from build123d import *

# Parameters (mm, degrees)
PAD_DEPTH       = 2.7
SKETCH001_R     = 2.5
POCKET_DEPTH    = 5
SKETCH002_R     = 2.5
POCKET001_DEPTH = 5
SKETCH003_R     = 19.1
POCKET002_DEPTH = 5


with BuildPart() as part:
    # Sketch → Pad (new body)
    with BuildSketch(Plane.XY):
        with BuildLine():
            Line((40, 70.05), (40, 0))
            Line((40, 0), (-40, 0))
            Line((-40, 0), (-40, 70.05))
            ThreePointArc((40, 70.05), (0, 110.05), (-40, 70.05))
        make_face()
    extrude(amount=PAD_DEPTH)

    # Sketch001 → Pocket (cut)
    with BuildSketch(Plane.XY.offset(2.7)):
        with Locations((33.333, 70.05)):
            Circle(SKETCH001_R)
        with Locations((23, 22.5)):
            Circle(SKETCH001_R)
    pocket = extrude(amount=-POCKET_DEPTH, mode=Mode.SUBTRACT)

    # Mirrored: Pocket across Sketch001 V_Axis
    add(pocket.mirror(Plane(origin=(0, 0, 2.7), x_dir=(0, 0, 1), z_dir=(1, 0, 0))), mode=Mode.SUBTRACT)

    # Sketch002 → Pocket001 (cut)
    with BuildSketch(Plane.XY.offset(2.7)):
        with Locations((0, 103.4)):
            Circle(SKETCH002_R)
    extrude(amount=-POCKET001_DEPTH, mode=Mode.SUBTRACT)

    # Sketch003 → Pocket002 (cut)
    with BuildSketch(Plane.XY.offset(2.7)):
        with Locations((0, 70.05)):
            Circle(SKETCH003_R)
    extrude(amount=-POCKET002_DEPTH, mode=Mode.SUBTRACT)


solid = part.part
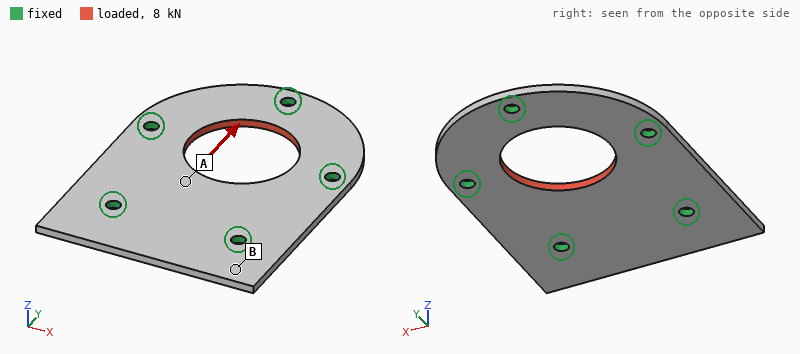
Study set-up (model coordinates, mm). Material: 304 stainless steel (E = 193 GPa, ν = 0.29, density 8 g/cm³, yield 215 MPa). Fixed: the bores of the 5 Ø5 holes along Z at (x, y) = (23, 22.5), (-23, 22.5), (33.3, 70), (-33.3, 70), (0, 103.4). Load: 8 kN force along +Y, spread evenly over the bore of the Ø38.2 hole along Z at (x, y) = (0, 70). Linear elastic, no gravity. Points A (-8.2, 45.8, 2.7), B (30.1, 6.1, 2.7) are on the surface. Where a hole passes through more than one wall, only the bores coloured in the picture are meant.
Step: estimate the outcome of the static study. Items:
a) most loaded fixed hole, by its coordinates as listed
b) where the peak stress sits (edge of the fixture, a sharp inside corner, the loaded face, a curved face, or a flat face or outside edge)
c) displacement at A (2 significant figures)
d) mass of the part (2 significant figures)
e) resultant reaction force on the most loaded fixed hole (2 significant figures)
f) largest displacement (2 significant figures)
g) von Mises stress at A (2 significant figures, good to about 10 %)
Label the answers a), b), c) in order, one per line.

a) (0, 103.4)
b) edge of the fixture
c) 3.6 µm
d) 150 g
e) 2.0 kN
f) 5.6 µm
g) 25 MPa
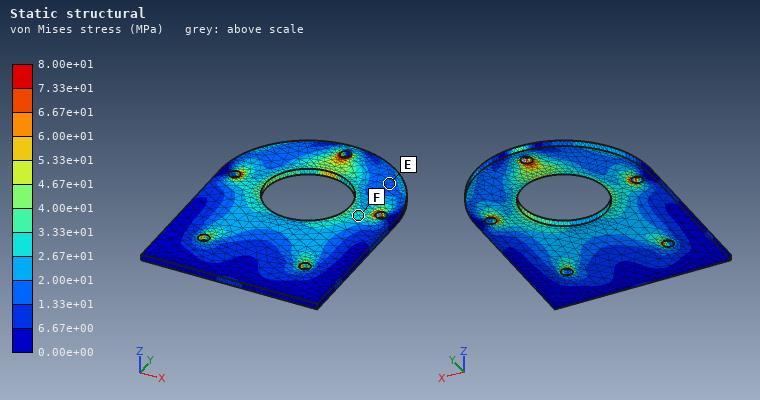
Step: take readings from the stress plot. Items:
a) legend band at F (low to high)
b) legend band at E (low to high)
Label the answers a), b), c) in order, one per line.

a) 2.67e+01 to 3.33e+01 MPa
b) 1.33e+01 to 2.00e+01 MPa
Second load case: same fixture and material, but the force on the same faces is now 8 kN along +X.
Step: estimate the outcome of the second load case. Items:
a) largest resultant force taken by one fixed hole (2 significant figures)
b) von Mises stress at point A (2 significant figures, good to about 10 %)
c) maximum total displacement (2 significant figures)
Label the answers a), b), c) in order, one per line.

a) 2.2 kN
b) 20 MPa
c) 6.3 µm
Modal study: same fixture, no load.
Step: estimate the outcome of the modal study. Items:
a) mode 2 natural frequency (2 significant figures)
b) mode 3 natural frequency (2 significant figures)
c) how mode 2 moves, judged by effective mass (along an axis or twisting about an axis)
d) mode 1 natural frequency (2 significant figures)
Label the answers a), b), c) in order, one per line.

a) 4100 Hz
b) 4500 Hz
c) along Z
d) 3600 Hz
